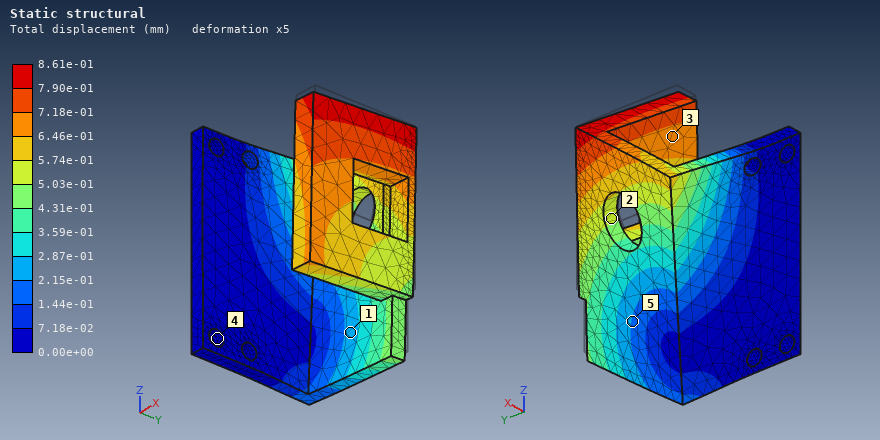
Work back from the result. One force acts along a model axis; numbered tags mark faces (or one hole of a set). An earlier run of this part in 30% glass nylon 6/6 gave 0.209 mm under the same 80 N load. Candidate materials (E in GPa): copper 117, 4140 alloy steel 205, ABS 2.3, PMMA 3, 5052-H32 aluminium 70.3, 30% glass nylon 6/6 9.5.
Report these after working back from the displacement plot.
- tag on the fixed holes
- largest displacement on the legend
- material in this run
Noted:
4
8.61e-01 mm
ABS
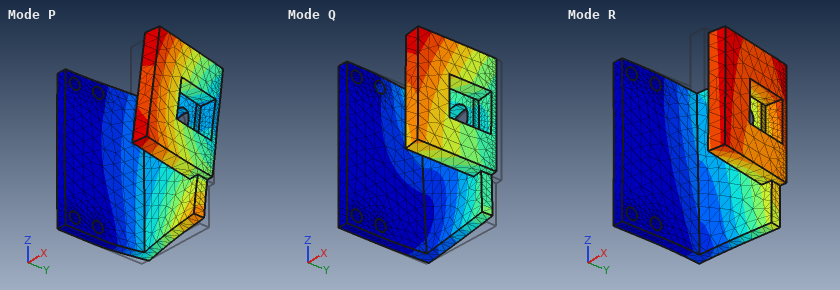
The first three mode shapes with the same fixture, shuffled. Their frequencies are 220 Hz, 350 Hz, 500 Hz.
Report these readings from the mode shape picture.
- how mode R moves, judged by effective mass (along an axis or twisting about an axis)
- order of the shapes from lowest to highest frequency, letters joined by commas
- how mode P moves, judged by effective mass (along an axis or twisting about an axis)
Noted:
along Y
R, Q, P
along X
